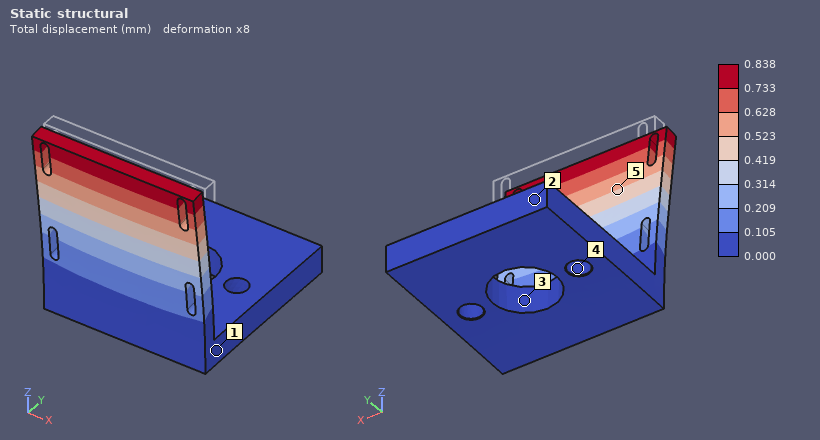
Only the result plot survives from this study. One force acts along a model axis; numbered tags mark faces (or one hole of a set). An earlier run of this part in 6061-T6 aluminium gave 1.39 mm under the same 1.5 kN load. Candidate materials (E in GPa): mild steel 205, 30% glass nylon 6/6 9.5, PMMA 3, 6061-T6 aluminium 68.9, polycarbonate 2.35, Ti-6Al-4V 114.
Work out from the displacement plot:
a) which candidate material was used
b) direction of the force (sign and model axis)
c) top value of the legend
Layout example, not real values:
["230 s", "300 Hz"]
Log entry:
["Ti-6Al-4V", "-Y", "0.838 mm"]
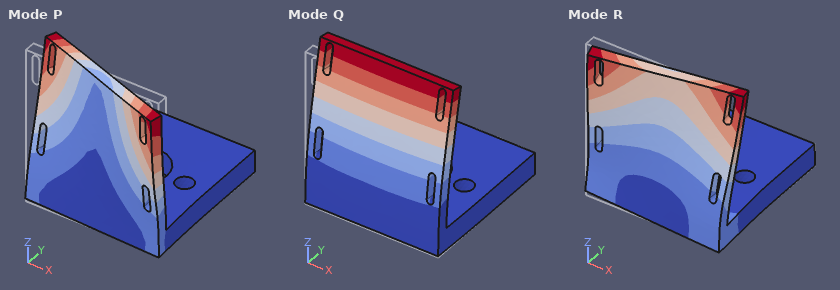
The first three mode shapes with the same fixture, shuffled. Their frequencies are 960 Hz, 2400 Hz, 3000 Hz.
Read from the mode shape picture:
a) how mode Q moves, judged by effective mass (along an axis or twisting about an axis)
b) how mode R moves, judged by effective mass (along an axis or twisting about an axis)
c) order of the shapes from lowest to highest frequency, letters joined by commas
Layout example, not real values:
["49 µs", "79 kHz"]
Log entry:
["along Y", "along X", "Q, P, R"]
